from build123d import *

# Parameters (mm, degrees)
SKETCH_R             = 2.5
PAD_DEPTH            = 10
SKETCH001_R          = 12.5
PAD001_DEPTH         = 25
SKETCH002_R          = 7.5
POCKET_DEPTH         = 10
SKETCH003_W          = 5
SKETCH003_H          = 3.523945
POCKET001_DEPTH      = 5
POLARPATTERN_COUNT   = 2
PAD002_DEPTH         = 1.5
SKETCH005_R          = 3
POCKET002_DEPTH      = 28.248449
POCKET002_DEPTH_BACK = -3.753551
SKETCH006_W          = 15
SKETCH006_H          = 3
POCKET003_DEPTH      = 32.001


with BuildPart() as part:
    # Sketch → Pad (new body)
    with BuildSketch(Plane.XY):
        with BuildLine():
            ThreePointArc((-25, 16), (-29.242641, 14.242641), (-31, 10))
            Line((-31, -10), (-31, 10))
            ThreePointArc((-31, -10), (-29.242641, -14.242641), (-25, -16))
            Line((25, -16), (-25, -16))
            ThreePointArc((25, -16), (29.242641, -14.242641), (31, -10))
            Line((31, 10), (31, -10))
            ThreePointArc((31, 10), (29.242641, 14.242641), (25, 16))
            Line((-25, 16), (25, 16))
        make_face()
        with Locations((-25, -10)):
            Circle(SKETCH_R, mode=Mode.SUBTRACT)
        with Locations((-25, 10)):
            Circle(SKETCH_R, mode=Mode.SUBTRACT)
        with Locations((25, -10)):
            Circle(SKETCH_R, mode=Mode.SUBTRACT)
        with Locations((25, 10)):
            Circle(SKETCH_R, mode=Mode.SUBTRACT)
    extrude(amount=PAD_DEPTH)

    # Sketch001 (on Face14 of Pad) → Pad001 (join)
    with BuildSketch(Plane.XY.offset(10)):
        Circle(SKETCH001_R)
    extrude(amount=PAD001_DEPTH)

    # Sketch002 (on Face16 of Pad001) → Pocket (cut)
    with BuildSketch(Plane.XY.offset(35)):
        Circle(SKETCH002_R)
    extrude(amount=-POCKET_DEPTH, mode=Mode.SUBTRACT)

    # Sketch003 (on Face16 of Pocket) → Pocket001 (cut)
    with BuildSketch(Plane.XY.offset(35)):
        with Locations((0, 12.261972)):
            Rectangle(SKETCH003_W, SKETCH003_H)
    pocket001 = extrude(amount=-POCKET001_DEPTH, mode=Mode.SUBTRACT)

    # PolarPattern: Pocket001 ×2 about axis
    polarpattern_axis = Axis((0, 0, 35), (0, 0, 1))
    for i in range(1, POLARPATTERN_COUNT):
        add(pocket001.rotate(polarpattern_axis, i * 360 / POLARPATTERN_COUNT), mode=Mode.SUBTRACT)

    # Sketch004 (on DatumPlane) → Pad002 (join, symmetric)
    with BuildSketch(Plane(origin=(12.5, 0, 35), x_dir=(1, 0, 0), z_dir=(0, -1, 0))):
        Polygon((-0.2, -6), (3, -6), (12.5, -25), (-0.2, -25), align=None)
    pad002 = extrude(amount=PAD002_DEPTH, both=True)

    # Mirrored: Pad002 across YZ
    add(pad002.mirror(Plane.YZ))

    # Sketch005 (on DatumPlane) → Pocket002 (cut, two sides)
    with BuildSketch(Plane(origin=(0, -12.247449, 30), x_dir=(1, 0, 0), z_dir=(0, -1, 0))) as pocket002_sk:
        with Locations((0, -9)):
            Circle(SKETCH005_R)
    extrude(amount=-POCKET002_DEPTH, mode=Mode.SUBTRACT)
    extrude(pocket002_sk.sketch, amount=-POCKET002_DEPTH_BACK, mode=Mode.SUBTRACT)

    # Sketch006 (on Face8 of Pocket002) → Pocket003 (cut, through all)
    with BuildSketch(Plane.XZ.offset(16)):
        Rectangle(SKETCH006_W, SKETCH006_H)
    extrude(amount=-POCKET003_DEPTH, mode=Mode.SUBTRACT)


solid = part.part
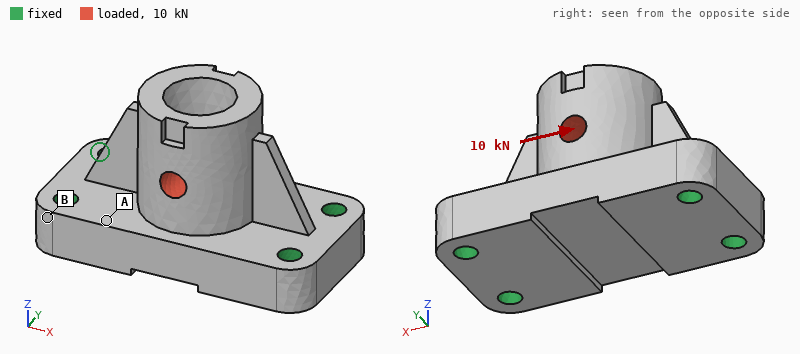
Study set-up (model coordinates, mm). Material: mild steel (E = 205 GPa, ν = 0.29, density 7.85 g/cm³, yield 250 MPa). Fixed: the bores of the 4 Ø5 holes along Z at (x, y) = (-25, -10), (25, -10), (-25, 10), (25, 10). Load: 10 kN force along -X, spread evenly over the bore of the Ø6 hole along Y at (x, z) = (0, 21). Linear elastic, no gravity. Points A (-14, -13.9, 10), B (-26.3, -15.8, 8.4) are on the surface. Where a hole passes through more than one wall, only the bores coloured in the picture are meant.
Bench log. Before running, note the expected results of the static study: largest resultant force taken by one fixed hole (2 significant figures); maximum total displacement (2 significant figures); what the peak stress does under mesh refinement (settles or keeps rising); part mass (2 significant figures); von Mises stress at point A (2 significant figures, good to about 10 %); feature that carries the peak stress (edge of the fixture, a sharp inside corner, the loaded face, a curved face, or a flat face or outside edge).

3.2 kN
12 µm
keeps rising
220 g
25 MPa
edge of the fixture
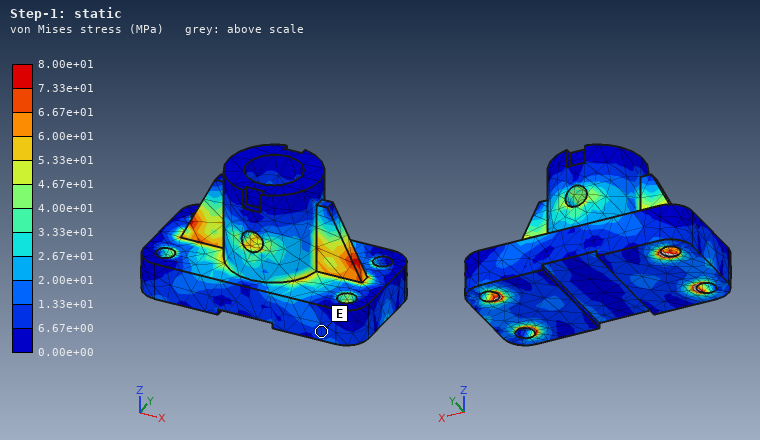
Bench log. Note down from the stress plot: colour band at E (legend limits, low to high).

6.67e+00 to 1.33e+01 MPa
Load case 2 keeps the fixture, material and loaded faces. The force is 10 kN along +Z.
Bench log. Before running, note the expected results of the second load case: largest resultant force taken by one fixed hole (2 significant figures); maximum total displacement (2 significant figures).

2.8 kN
11 µm
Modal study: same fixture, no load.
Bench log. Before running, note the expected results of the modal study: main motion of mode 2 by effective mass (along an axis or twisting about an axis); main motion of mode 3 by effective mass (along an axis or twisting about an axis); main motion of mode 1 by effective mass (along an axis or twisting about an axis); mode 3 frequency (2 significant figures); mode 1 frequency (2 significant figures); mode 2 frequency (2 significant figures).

along Z
along X
along Y
18 kHz
9000 Hz
15 kHz
